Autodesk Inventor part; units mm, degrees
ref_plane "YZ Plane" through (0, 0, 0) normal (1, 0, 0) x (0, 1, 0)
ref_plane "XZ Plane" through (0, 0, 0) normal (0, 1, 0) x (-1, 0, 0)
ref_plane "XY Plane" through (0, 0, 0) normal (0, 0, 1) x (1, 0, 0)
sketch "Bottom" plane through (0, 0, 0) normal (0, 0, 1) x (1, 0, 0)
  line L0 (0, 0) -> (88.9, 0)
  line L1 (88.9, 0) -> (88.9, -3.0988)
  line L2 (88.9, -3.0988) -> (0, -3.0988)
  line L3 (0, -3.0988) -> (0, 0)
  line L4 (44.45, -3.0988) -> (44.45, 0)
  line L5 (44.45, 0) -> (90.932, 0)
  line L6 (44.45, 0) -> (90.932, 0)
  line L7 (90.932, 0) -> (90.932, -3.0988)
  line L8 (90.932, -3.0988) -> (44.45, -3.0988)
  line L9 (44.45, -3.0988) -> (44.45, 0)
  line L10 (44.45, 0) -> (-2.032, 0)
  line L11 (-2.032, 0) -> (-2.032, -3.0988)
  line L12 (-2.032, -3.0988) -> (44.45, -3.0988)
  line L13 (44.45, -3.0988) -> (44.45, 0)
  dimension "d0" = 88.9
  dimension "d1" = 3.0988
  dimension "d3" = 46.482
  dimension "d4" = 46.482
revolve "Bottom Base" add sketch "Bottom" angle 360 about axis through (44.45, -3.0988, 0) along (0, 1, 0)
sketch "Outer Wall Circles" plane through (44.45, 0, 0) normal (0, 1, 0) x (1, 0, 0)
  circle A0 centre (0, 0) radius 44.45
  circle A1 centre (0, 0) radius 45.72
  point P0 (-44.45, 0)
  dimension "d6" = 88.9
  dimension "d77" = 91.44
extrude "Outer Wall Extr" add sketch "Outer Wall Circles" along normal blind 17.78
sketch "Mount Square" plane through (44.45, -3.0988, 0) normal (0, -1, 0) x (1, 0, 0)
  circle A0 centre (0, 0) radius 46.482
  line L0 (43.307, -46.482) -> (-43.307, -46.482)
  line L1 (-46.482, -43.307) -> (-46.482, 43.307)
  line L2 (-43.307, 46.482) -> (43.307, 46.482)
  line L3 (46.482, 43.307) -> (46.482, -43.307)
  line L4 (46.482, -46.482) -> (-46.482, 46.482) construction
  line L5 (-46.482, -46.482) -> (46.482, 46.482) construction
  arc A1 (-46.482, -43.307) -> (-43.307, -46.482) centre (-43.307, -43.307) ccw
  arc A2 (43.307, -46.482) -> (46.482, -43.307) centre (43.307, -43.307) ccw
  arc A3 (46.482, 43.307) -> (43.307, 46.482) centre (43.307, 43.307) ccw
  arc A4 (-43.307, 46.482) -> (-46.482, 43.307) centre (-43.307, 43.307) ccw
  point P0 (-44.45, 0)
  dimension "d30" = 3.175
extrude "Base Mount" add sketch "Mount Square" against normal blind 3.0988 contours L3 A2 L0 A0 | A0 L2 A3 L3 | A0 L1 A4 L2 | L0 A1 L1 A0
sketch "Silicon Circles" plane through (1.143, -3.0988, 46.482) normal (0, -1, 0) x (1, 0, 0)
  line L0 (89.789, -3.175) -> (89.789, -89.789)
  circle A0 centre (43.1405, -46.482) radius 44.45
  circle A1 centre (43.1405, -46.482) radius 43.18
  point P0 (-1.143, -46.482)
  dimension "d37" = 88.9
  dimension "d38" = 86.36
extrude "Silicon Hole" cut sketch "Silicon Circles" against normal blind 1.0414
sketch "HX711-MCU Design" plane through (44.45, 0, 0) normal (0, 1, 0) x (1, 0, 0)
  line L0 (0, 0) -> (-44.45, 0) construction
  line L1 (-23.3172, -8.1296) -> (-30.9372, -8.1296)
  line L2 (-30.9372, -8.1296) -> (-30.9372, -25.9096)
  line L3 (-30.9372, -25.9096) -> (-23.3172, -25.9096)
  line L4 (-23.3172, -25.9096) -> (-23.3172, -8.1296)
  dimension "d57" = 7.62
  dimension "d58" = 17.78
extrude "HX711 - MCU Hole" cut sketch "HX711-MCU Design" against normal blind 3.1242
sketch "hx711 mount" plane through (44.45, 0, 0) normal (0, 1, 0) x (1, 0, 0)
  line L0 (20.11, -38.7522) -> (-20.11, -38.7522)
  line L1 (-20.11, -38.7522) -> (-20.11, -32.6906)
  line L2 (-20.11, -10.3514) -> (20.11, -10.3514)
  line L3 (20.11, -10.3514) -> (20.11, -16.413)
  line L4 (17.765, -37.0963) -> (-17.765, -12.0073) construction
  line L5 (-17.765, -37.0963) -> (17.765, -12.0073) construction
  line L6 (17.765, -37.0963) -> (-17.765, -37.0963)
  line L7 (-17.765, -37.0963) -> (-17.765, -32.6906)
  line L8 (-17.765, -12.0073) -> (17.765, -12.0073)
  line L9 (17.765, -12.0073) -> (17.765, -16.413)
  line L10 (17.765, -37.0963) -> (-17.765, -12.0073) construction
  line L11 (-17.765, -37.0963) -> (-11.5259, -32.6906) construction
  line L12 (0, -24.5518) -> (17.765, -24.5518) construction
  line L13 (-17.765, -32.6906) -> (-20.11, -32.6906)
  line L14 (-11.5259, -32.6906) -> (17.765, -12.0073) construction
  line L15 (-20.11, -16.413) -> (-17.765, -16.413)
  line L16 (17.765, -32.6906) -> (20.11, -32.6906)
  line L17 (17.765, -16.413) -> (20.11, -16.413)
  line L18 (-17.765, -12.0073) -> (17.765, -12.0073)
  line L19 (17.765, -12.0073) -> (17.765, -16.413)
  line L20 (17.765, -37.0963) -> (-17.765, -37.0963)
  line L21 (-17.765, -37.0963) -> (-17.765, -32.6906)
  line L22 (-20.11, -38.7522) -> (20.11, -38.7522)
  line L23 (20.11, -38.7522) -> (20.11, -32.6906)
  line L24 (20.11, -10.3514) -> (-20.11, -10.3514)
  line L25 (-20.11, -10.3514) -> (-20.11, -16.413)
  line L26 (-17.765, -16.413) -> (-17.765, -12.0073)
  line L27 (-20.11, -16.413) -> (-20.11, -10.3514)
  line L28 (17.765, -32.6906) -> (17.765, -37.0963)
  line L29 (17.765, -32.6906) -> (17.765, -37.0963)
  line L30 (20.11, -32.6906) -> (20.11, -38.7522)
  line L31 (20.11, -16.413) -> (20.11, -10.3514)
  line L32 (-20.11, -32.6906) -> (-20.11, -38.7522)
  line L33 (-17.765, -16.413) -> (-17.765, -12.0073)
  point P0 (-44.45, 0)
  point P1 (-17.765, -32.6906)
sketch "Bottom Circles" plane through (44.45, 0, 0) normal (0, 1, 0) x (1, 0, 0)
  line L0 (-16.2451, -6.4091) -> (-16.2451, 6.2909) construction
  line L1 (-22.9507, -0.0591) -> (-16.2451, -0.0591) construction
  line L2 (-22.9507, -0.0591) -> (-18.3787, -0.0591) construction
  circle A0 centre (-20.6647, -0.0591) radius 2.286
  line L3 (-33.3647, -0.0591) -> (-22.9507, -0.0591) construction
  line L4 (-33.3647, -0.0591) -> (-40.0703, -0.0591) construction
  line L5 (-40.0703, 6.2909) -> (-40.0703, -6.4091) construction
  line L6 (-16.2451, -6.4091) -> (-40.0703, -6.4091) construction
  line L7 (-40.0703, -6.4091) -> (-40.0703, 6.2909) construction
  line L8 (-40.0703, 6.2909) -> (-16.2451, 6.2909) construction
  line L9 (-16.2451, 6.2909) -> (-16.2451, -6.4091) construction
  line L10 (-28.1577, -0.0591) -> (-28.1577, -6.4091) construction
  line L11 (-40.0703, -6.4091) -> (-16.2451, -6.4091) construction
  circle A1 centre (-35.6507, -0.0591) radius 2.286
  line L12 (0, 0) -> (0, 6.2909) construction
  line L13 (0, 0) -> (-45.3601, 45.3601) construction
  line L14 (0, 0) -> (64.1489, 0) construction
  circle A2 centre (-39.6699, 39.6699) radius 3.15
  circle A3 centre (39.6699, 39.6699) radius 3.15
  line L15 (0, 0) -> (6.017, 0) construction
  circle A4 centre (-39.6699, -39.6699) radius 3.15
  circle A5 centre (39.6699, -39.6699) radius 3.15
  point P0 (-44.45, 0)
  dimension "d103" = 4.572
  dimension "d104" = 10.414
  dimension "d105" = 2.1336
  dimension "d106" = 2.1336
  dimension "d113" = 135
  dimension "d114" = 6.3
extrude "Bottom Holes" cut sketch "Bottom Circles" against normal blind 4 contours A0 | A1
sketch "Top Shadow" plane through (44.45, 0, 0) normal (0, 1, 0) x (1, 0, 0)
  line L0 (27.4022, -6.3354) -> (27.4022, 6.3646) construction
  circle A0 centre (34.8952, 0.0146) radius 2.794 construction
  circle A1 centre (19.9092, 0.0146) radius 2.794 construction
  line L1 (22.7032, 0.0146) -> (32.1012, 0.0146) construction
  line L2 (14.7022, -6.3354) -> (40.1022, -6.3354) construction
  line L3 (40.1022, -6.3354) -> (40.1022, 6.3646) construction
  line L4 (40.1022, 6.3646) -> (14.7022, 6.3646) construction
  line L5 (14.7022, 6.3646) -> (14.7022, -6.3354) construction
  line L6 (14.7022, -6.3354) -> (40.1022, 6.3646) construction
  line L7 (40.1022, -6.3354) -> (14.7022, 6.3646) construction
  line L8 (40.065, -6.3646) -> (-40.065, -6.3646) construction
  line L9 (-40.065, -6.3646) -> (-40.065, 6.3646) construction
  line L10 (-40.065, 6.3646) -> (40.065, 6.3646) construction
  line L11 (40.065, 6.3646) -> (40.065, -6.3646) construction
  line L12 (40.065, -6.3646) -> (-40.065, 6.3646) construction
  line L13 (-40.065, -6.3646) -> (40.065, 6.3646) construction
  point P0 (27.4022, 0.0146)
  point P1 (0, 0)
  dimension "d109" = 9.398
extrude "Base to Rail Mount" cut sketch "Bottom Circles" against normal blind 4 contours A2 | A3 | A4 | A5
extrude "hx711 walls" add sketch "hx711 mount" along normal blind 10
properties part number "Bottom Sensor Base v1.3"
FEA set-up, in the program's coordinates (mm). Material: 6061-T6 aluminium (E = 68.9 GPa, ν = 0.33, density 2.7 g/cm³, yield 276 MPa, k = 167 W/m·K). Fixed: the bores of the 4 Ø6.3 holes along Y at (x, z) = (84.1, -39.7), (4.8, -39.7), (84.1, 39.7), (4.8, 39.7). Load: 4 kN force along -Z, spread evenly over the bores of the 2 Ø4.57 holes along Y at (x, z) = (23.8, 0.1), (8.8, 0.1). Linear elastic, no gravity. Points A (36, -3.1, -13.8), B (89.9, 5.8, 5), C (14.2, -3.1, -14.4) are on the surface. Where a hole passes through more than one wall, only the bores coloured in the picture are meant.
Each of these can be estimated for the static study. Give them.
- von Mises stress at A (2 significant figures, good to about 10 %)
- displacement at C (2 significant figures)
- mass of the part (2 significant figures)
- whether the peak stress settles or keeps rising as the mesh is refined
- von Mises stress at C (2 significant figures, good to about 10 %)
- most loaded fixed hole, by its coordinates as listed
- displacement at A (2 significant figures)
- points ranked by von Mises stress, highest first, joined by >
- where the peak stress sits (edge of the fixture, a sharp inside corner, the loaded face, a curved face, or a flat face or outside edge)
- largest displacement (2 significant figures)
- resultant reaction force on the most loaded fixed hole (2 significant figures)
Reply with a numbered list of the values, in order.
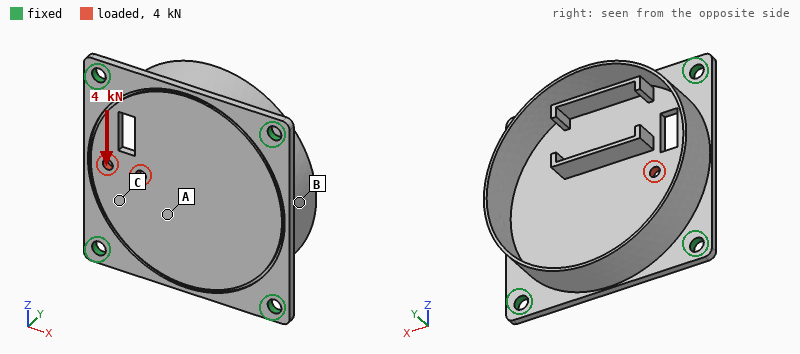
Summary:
1. 9.2 MPa
2. 12 µm
3. 91 g
4. keeps rising
5. 22 MPa
6. (4.8, -39.7)
7. 10 µm
8. C > A > B
9. edge of the fixture
10. 18 µm
11. 1.7 kN
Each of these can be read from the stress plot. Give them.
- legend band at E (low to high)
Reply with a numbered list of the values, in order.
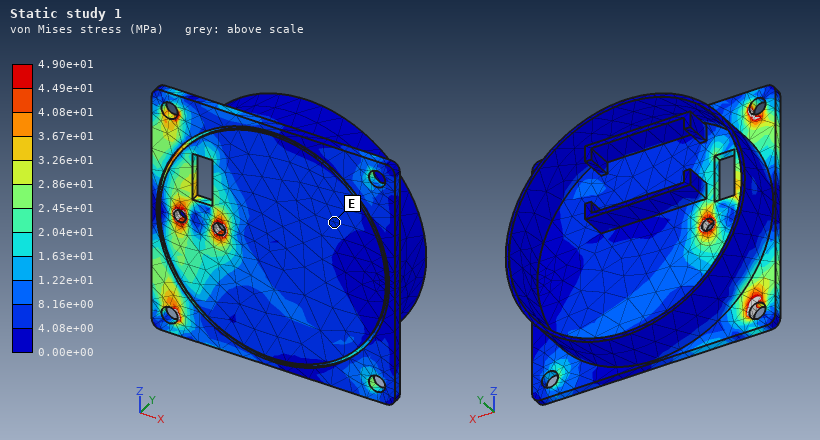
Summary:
1. 4.08e+00 to 8.16e+00 MPa
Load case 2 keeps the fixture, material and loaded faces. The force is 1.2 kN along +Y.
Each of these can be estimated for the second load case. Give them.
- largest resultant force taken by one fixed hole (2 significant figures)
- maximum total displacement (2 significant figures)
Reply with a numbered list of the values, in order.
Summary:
1. 620 N
2. 0.34 mm
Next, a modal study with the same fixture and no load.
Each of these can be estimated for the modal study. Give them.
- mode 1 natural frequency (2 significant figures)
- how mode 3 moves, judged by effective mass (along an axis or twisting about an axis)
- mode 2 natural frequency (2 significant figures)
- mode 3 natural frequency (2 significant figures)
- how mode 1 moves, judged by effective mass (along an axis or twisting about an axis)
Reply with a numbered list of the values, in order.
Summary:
1. 2100 Hz
2. twisting about Z
3. 3000 Hz
4. 3200 Hz
5. along Y
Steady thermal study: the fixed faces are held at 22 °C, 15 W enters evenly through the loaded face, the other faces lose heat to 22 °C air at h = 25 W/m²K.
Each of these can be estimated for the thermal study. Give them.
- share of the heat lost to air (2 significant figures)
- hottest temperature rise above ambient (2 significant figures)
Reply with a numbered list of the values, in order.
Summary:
1. 20 %
2. 15 K
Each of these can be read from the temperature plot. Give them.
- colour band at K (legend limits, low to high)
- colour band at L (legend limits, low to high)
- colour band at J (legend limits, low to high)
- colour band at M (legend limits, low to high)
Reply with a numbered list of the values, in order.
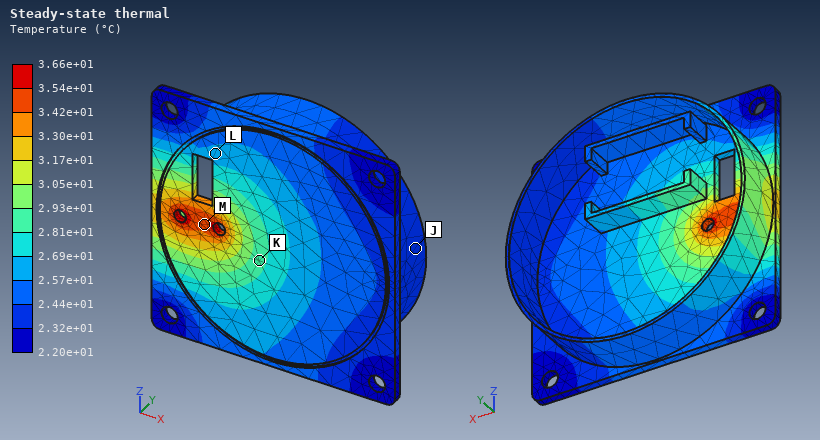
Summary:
1. 2.81e+01 to 2.93e+01 °C
2. 2.57e+01 to 2.69e+01 °C
3. 2.32e+01 to 2.44e+01 °C
4. 3.42e+01 to 3.54e+01 °C
